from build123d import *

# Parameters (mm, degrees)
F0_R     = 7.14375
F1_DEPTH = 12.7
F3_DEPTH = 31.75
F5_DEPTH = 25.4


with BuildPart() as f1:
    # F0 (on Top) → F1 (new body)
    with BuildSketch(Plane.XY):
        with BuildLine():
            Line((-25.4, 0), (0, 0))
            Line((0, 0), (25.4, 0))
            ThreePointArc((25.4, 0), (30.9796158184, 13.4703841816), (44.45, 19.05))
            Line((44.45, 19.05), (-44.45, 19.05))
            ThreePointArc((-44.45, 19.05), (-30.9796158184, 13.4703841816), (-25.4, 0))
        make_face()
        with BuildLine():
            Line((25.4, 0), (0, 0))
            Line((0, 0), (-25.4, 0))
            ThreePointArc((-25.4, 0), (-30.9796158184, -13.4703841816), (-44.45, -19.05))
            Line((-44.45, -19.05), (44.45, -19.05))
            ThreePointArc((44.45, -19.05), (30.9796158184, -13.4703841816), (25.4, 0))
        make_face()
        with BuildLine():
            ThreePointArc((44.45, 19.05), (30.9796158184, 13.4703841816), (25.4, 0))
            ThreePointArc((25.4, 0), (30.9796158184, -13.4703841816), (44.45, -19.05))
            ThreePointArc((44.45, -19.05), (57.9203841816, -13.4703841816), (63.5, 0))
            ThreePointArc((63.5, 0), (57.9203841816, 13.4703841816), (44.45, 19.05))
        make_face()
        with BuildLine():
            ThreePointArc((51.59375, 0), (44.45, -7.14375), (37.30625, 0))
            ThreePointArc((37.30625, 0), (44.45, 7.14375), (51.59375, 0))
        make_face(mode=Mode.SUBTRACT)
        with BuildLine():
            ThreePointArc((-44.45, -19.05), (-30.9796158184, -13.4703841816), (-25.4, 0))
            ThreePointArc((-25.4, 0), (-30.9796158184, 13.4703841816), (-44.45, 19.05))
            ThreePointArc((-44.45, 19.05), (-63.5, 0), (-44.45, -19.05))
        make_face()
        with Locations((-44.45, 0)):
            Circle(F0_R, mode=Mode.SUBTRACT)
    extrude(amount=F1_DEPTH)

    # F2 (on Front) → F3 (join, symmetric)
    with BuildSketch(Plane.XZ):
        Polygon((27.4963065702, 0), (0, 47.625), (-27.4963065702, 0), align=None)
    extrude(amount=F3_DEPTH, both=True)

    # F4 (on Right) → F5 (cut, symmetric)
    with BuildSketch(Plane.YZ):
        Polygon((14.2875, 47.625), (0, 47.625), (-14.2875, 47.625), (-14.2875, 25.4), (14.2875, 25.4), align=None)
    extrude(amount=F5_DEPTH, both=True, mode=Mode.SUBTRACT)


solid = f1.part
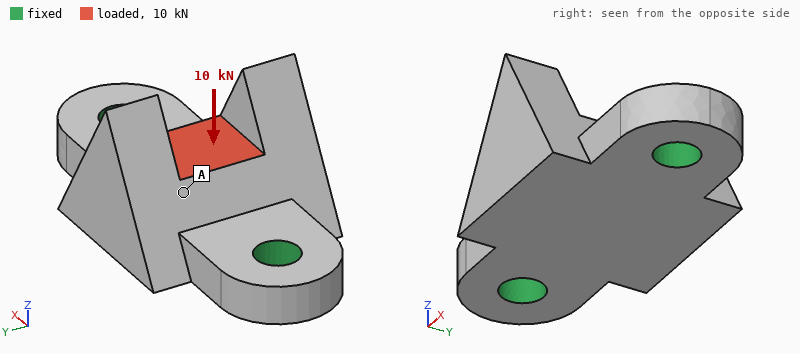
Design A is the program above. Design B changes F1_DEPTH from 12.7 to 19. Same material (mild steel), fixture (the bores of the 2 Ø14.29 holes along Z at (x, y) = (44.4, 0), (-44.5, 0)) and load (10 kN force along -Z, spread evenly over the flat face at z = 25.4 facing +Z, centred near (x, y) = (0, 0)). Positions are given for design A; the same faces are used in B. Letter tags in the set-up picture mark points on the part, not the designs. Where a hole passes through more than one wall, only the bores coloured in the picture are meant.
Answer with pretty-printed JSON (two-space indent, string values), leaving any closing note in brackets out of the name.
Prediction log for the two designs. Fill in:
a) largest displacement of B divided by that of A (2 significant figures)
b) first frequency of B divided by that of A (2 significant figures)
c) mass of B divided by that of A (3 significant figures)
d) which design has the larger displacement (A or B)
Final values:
{
  "largest displacement of B divided by that of A": "0.61",
  "first frequency of B divided by that of A": "1.5",
  "mass of B divided by that of A": "1.17",
  "which design has the larger displacement": "A"
}
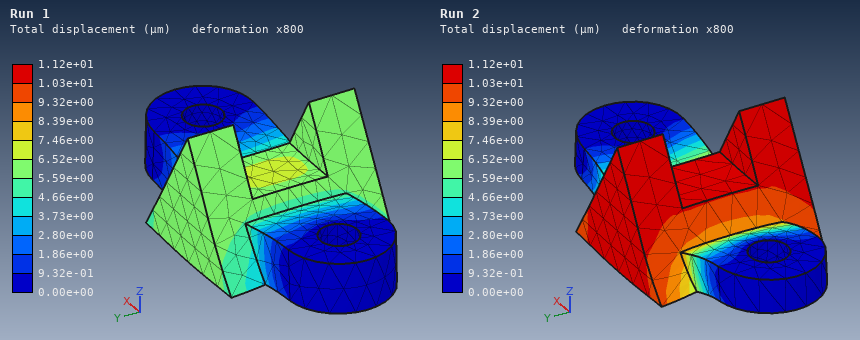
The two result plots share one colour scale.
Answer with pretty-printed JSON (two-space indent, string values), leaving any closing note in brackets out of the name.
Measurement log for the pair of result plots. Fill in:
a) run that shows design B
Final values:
{
  "run that shows design B": "Run 1"
}
